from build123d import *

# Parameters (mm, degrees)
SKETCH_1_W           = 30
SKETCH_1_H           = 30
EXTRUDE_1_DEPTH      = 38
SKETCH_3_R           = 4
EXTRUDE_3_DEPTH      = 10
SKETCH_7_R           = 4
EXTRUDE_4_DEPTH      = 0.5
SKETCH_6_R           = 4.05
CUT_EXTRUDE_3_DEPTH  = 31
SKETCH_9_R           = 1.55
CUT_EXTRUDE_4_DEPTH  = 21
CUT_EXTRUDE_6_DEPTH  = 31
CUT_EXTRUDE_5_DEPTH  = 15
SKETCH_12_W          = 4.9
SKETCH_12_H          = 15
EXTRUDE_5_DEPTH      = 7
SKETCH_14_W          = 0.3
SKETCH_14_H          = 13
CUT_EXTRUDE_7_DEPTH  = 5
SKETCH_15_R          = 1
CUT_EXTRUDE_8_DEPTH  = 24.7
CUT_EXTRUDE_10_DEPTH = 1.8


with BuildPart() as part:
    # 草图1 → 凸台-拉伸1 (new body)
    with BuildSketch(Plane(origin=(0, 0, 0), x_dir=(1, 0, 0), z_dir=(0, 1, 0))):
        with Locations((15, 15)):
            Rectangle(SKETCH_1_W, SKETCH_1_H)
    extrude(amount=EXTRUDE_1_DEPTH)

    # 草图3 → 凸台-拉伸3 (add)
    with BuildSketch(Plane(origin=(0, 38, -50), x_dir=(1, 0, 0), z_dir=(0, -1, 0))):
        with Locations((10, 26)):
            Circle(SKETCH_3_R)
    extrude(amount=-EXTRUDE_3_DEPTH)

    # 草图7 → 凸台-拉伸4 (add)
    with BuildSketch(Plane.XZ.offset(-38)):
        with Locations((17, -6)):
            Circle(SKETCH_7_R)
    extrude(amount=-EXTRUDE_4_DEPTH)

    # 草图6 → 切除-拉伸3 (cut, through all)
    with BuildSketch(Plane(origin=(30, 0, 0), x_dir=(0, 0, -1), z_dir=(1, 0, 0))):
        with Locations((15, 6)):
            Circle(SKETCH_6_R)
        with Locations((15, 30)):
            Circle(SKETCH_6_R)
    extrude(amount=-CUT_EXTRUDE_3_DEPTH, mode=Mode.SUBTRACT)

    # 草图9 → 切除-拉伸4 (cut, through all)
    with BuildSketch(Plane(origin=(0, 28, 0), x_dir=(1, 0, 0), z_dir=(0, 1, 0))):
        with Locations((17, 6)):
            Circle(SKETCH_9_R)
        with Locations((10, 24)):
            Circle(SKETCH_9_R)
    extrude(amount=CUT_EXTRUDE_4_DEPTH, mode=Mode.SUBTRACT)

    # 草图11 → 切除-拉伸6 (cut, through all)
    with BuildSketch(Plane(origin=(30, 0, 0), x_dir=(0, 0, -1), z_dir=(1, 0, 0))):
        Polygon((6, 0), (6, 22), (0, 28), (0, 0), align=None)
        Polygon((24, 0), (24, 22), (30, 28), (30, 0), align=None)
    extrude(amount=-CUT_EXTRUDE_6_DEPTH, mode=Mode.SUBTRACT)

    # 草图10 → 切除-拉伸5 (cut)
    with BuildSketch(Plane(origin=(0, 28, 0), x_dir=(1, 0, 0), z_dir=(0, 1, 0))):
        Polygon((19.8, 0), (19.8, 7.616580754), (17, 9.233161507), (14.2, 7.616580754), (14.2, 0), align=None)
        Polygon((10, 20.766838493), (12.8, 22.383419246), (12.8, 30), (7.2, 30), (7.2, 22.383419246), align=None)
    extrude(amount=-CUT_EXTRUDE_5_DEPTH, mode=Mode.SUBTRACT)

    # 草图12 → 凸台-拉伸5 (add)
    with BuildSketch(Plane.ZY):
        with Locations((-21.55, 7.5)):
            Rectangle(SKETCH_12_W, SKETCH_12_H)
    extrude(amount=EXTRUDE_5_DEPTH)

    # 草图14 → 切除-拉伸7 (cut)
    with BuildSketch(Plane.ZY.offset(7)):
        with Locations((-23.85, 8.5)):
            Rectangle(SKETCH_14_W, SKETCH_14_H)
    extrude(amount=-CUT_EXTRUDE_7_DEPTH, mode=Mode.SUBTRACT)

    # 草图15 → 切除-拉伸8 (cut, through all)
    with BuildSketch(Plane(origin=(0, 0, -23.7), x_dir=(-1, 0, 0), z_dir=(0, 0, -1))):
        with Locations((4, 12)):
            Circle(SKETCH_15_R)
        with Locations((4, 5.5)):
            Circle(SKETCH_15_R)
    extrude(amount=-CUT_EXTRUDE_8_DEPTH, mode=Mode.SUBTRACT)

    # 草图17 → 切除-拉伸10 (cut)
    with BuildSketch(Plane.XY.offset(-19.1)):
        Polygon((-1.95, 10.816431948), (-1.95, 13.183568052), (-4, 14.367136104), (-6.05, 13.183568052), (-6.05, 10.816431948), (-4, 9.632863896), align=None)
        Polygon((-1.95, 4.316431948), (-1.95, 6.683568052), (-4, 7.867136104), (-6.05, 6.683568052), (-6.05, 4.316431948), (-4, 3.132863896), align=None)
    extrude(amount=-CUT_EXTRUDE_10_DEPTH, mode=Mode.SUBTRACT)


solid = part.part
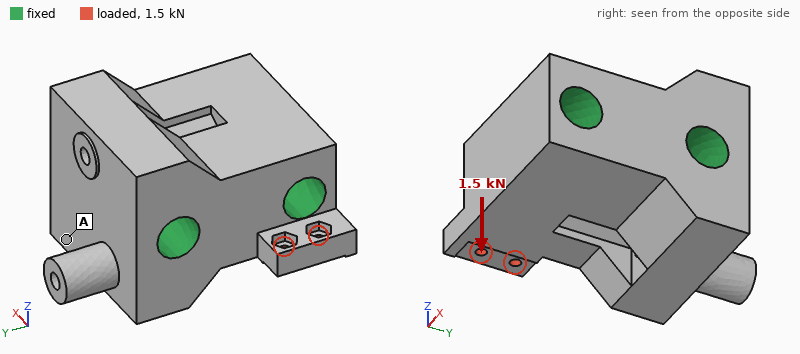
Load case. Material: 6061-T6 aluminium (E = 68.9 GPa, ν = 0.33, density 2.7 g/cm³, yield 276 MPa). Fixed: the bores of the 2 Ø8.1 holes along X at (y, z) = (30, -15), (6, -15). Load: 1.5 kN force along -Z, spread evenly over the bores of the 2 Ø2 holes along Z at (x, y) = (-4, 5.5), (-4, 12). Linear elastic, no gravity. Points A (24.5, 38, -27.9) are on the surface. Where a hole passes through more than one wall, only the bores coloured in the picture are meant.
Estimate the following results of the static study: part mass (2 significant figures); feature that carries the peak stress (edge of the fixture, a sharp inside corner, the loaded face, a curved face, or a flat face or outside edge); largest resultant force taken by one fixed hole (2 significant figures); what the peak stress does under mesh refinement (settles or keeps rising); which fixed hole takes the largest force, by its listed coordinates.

60 g
edge of the fixture
1.4 kN
keeps rising
(6, -15)
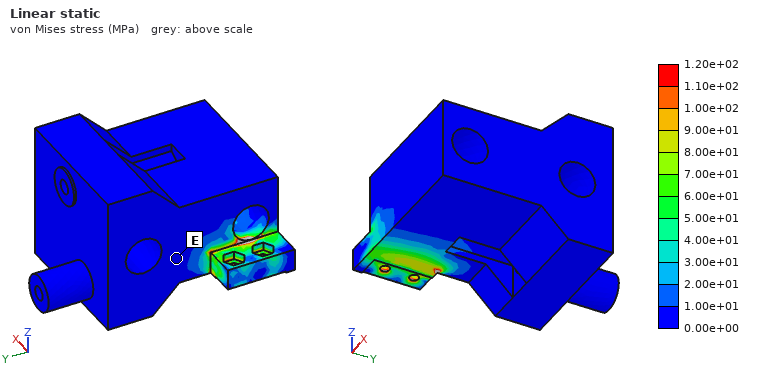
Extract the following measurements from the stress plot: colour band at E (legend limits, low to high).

0.00e+00 to 1.00e+01 MPa
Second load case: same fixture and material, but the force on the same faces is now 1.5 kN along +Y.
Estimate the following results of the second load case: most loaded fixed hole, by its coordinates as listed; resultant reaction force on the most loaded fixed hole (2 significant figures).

(6, -15)
1.2 kN
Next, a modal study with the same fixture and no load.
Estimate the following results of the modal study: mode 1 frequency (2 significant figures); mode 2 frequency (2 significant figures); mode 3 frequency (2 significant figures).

31 kHz
33 kHz
42 kHz
